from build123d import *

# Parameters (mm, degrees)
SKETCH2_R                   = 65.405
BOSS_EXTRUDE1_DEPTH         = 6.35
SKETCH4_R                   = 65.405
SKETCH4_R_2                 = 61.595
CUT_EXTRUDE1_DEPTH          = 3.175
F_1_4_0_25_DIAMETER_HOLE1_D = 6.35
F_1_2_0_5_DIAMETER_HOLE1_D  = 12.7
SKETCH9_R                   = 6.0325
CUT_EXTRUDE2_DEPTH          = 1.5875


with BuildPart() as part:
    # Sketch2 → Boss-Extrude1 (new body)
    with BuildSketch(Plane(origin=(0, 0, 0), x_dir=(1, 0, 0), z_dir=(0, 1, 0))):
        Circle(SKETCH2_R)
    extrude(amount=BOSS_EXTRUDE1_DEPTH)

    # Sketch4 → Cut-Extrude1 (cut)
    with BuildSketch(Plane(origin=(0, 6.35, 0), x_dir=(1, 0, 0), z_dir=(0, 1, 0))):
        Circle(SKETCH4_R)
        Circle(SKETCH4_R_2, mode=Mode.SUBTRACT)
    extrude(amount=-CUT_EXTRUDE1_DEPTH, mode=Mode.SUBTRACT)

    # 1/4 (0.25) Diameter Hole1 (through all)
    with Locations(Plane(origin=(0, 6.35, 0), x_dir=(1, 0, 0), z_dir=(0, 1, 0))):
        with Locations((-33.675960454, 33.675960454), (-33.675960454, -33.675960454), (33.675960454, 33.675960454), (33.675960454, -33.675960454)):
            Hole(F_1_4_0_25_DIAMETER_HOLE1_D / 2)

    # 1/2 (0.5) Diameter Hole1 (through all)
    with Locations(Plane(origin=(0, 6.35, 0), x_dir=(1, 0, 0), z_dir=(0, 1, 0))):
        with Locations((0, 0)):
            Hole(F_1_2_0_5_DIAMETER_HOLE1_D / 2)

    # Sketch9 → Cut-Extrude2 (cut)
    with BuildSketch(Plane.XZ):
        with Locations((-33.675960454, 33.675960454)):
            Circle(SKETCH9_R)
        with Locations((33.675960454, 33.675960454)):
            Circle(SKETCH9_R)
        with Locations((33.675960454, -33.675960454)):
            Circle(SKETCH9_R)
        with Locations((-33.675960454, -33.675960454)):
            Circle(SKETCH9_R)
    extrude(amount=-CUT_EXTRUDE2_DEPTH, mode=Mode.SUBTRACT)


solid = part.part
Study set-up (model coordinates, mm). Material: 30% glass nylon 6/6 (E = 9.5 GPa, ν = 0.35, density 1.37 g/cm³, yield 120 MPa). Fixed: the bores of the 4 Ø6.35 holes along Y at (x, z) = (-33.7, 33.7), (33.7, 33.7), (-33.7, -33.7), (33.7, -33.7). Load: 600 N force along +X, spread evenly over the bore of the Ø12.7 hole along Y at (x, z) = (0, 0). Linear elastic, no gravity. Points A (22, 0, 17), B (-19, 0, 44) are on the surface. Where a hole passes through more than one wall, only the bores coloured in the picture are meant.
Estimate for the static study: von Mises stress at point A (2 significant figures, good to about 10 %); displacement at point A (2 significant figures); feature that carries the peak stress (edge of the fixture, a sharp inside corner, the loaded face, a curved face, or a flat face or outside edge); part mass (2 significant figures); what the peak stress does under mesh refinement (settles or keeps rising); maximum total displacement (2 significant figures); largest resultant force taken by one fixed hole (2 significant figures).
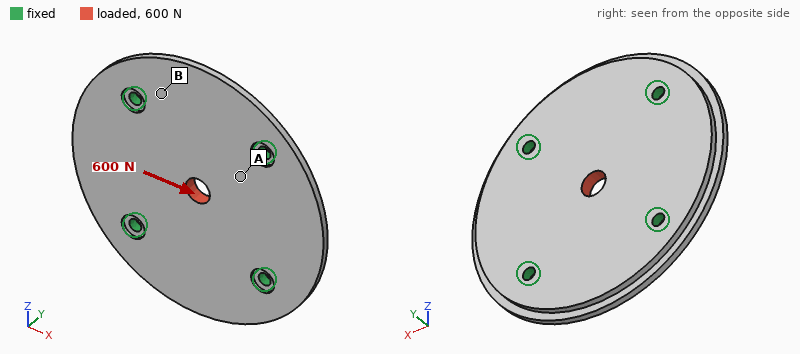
0.98 MPa
3.2 µm
edge of the fixture
110 g
keeps rising
7.4 µm
160 N
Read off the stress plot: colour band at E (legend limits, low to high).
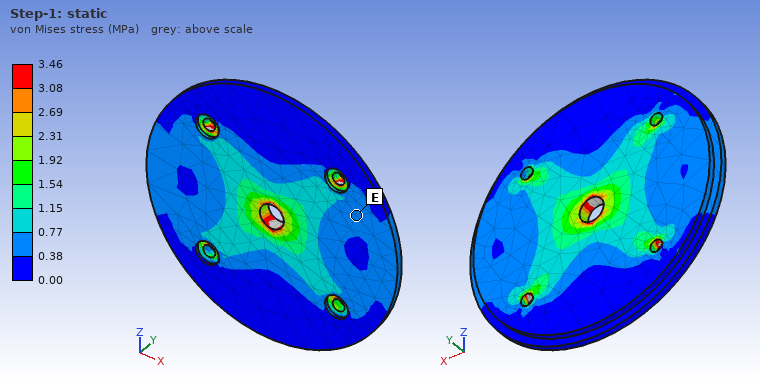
0.38 to 0.77 MPa
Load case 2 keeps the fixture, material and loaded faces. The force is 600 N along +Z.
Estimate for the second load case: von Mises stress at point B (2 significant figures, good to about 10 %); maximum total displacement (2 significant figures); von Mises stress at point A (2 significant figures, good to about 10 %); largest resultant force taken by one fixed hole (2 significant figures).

0.51 MPa
7.4 µm
0.94 MPa
160 N
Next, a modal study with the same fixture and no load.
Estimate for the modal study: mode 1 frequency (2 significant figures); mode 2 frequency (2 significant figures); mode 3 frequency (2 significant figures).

2000 Hz
2200 Hz
2200 Hz
